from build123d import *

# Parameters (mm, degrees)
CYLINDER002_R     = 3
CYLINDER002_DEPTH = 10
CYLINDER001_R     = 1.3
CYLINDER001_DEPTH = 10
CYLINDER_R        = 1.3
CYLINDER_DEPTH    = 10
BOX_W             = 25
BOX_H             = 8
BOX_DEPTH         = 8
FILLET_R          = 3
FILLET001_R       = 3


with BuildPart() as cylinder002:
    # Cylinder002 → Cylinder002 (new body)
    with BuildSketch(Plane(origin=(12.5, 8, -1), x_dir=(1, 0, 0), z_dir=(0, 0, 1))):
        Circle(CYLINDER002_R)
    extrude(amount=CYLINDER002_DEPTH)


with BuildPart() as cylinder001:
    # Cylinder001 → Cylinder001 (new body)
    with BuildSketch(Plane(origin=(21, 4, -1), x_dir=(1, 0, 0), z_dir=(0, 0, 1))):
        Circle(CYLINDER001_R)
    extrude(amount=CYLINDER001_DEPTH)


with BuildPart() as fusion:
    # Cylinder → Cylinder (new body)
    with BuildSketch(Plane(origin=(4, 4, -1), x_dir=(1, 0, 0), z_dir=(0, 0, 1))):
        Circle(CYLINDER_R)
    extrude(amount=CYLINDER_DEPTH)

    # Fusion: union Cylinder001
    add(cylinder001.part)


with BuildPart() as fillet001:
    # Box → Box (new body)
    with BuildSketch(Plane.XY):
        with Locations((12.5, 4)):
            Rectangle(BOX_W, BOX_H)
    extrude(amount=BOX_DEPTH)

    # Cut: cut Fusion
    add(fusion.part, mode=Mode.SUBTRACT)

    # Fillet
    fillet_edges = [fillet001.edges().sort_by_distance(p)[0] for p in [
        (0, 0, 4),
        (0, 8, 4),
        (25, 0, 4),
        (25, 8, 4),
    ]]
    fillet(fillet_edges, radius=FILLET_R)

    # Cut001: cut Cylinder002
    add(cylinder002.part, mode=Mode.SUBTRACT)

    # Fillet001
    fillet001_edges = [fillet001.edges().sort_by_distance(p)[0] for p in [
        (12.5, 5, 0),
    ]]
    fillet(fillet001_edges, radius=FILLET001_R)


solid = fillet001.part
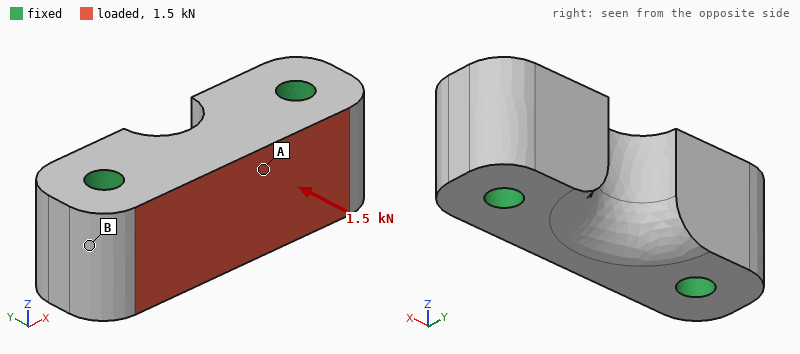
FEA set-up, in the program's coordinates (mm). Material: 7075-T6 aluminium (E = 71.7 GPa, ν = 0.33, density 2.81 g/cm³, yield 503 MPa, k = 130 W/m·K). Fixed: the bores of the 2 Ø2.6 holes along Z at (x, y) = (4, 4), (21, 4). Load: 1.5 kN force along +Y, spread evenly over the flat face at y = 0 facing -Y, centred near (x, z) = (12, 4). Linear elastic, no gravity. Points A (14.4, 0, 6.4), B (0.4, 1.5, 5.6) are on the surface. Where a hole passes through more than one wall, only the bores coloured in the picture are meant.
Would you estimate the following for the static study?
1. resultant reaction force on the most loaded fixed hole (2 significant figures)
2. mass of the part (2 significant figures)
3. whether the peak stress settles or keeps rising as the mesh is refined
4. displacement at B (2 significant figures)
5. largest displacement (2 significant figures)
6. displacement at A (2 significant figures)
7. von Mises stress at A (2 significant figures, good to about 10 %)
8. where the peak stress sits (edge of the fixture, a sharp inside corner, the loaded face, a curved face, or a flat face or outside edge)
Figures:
810 N
3.7 g
keeps rising
0.78 µm
4.3 µm
3.7 µm
22 MPa
edge of the fixture
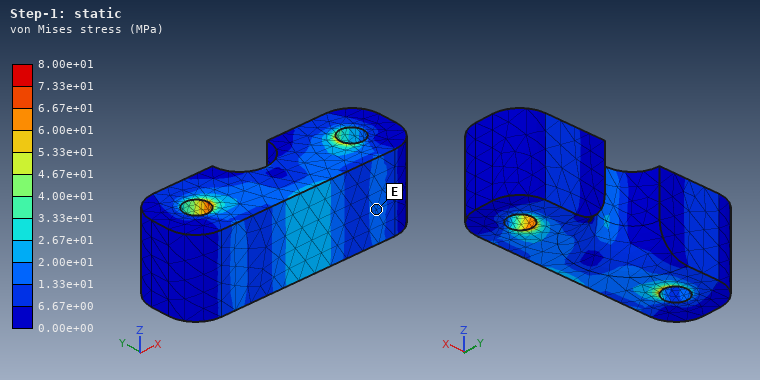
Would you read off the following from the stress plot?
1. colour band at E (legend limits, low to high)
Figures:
1.33e+01 to 2.00e+01 MPa
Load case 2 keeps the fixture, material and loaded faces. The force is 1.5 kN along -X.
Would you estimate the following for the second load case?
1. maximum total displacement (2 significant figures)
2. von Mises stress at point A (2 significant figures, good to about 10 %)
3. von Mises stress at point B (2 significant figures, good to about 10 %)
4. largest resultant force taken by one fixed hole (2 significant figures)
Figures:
1.7 µm
17 MPa
4.5 MPa
800 N
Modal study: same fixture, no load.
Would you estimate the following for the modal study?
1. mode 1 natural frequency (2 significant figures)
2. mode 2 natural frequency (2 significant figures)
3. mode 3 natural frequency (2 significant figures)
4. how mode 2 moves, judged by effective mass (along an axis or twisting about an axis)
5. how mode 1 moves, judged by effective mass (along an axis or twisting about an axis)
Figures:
66 kHz
79 kHz
110 kHz
along Z
along Y
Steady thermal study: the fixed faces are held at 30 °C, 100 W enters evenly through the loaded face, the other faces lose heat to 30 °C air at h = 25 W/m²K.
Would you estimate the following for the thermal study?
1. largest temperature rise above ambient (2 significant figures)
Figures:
37 K
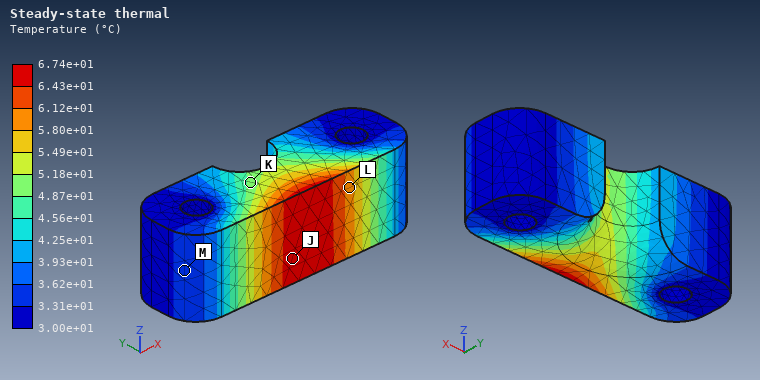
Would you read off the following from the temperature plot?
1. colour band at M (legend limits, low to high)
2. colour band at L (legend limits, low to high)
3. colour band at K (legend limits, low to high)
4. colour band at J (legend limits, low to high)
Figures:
3.31e+01 to 3.62e+01 °C
5.80e+01 to 6.12e+01 °C
4.87e+01 to 5.18e+01 °C
6.43e+01 to 6.74e+01 °C
